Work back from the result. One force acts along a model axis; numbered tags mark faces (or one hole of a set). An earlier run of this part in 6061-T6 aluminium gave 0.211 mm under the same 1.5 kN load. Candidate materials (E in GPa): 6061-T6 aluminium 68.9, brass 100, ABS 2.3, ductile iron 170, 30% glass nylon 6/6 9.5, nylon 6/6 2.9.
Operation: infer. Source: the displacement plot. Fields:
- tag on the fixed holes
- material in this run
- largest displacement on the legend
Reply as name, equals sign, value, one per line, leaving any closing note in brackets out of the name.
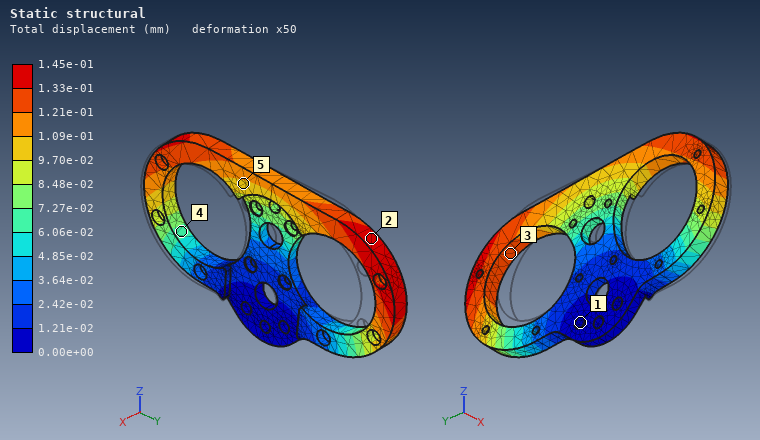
tag on the fixed holes = 1
material in this run = brass
largest displacement on the legend = 1.45e-01 mm
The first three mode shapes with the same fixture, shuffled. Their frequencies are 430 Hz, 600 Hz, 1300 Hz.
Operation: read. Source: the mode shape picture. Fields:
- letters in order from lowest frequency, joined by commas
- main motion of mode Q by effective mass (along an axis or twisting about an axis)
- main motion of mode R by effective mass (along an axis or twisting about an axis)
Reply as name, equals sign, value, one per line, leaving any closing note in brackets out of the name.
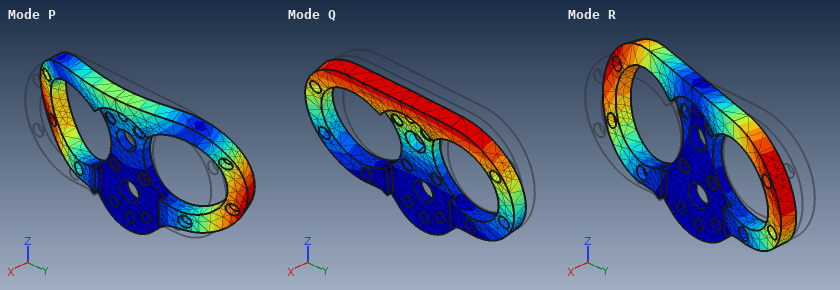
letters in order from lowest frequency, joined by commas = Q, R, P
main motion of mode Q by effective mass = along X
main motion of mode R by effective mass = twisting about Z
